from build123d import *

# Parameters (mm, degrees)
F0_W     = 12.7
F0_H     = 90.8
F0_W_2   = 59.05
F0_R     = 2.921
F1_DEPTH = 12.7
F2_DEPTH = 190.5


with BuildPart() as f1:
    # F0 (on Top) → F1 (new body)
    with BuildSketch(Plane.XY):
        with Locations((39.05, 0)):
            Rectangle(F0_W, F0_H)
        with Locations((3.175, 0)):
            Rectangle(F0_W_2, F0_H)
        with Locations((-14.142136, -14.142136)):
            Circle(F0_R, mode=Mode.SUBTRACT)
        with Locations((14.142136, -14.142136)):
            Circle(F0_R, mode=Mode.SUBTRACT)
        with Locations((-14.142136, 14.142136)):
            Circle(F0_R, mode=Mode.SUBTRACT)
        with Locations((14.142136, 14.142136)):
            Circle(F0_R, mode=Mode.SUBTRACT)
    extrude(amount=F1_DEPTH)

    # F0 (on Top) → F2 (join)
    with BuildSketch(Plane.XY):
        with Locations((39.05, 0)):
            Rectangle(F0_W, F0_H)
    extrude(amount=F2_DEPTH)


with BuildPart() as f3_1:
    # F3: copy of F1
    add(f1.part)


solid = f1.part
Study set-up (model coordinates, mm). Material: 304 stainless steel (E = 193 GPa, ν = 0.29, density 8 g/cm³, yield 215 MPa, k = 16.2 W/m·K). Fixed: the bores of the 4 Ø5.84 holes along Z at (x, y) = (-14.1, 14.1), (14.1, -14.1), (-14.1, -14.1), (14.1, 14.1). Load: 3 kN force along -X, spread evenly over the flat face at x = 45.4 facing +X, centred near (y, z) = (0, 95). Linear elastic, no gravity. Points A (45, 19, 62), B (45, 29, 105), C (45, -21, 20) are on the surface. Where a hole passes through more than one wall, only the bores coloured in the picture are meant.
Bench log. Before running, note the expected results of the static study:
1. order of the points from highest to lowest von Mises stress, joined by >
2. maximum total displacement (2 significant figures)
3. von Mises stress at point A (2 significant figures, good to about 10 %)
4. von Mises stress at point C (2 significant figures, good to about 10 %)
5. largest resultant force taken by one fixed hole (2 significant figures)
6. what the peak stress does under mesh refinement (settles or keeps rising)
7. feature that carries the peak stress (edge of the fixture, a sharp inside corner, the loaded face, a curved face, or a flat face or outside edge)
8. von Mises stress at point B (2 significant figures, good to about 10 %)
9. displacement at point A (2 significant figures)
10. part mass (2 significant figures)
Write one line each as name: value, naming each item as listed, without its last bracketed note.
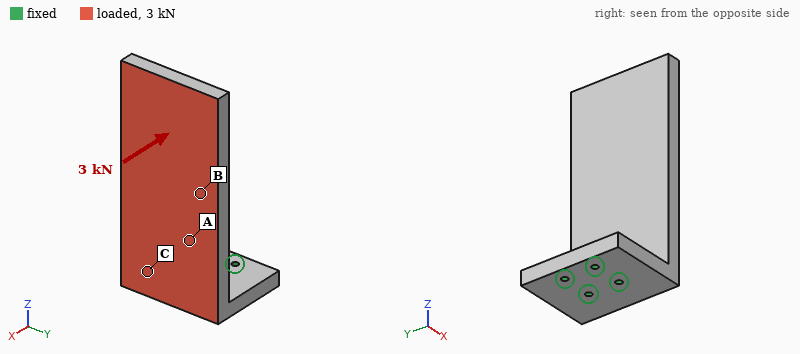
order of the points from highest to lowest von Mises stress, joined by >: C > A > B
maximum total displacement: 1.1 mm
von Mises stress at point A: 51 MPa
von Mises stress at point C: 83 MPa
largest resultant force taken by one fixed hole: 2.5 kN
what the peak stress does under mesh refinement: keeps rising
feature that carries the peak stress: edge of the fixture
von Mises stress at point B: 24 MPa
displacement at point A: 0.23 mm
part mass: 2.3 kg
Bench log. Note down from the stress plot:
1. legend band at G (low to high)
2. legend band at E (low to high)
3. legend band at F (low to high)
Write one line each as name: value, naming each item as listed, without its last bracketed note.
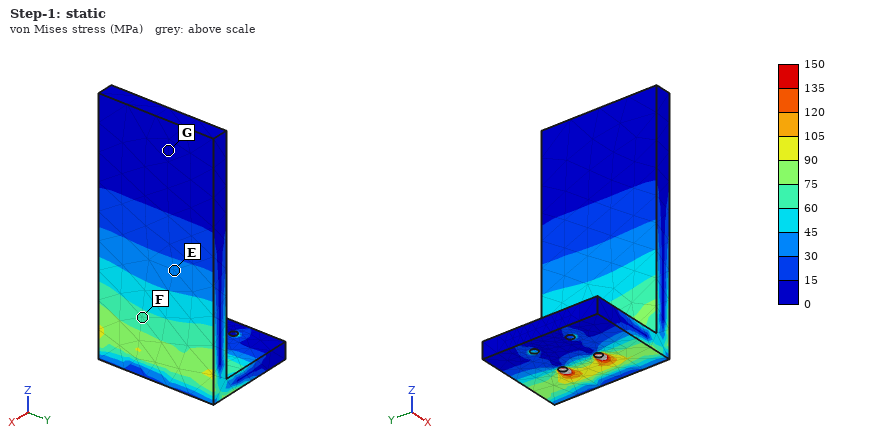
legend band at G: 0 to 15 MPa
legend band at E: 30 to 45 MPa
legend band at F: 60 to 75 MPa
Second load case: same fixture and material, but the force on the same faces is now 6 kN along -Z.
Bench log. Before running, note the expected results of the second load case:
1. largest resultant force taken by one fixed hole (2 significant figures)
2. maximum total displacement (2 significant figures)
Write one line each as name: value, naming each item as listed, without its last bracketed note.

largest resultant force taken by one fixed hole: 4.2 kN
maximum total displacement: 0.34 mm
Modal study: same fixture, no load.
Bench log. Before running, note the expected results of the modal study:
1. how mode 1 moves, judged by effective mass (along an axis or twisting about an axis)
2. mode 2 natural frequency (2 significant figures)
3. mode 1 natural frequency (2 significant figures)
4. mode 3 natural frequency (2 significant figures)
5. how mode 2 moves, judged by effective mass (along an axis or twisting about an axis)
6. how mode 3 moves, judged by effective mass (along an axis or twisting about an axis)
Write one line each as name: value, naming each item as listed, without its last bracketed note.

how mode 1 moves, judged by effective mass: along X
mode 2 natural frequency: 610 Hz
mode 1 natural frequency: 240 Hz
mode 3 natural frequency: 1200 Hz
how mode 2 moves, judged by effective mass: along Y
how mode 3 moves, judged by effective mass: twisting about Z
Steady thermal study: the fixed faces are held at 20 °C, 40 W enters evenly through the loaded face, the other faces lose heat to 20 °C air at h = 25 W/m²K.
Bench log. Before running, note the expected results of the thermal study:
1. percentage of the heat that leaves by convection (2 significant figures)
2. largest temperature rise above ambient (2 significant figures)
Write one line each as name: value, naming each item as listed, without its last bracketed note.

percentage of the heat that leaves by convection: 70 %
largest temperature rise above ambient: 58 K
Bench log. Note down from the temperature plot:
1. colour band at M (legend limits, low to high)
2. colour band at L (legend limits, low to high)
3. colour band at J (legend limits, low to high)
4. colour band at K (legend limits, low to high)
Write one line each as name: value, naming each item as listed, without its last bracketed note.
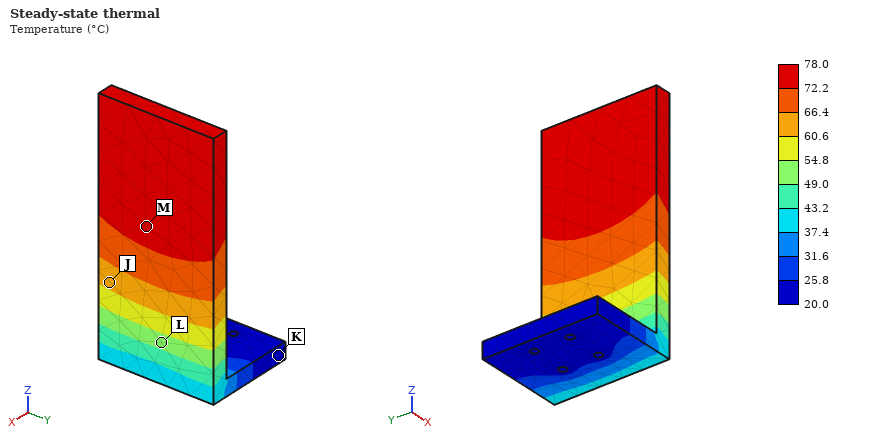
colour band at M: 72.2 to 78.0 °C
colour band at L: 49.0 to 54.8 °C
colour band at J: 60.6 to 66.4 °C
colour band at K: 20.0 to 25.8 °C
